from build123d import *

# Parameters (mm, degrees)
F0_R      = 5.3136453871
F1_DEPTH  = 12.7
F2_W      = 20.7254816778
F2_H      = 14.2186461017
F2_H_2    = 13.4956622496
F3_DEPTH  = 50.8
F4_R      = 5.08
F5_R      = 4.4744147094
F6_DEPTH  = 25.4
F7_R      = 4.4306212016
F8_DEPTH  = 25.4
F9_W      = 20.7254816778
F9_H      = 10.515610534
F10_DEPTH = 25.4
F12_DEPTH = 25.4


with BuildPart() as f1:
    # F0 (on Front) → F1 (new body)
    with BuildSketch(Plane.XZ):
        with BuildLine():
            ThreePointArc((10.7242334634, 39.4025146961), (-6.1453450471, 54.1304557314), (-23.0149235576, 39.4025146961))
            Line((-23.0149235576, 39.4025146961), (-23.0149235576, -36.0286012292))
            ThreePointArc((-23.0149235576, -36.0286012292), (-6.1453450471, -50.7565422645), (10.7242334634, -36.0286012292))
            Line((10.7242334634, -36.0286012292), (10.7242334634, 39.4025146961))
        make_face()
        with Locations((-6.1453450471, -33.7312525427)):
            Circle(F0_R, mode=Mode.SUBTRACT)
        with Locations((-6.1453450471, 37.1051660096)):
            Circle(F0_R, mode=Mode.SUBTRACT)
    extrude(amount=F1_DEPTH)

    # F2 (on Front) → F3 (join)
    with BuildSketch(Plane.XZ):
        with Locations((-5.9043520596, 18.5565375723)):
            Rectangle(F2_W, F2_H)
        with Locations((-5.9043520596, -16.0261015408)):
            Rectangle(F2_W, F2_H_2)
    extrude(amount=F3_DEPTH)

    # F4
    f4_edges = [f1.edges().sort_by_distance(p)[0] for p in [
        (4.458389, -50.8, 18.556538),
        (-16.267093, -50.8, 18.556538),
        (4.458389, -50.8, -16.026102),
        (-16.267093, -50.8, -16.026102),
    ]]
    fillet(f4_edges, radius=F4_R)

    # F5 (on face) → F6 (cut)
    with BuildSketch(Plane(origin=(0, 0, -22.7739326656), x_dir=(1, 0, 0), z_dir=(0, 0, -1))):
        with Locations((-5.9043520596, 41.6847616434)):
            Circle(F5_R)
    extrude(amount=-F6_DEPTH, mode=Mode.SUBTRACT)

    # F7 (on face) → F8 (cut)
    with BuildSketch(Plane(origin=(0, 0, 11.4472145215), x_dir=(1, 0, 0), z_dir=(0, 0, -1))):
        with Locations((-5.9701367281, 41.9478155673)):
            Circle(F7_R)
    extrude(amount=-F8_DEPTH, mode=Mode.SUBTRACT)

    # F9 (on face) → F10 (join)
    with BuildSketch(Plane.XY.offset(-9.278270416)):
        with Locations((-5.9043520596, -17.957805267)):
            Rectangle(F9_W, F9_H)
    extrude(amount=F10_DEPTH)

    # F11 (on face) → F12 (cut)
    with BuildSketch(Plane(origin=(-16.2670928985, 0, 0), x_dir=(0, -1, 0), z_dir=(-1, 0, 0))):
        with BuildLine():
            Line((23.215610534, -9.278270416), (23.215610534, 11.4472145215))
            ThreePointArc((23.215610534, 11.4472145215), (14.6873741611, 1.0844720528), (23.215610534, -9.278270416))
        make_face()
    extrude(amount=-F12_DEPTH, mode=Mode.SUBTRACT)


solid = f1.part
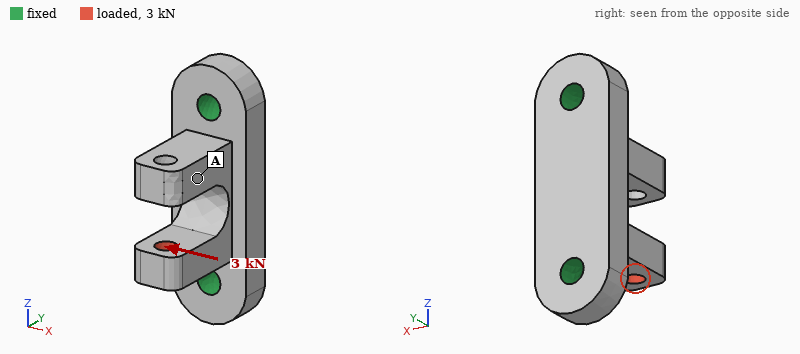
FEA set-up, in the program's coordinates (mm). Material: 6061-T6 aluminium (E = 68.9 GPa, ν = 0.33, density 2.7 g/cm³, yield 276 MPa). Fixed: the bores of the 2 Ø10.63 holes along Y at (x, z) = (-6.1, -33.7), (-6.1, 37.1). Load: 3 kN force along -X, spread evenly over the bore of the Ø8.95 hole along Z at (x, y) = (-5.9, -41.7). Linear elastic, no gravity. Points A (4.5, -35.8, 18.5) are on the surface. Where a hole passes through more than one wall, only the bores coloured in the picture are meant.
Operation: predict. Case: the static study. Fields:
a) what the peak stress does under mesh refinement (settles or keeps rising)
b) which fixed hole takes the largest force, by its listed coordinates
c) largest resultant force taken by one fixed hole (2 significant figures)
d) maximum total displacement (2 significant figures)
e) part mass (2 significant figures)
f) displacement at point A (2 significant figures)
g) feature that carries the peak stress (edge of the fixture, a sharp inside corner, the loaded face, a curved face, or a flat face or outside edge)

keeps rising
(-6.1, -33.7)
2.4 kN
0.16 mm
170 g
0.031 mm
edge of the fixture
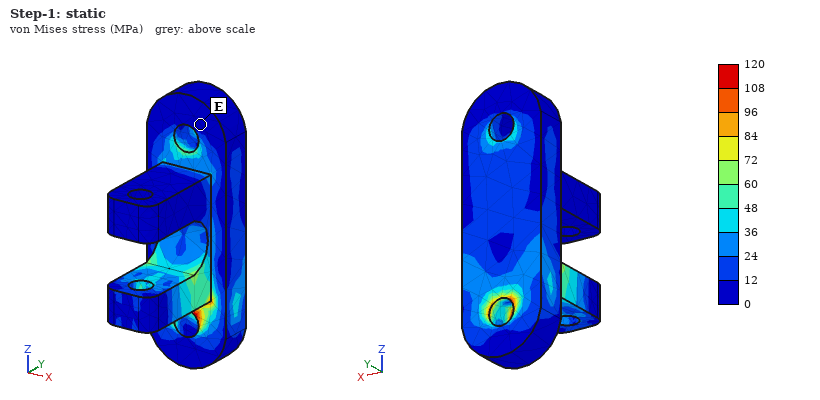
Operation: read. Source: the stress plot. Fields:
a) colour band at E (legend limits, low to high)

0 to 12 MPa
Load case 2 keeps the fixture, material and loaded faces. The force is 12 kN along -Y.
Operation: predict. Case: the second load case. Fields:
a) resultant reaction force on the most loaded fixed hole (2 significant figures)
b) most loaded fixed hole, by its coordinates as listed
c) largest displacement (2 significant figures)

9.9 kN
(-6.1, -33.7)
58 µm
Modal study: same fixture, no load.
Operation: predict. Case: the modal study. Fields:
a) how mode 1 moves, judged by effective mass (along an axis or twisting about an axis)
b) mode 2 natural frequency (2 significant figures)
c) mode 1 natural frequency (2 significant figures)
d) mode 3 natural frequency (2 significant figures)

along X
6400 Hz
5500 Hz
7900 Hz
